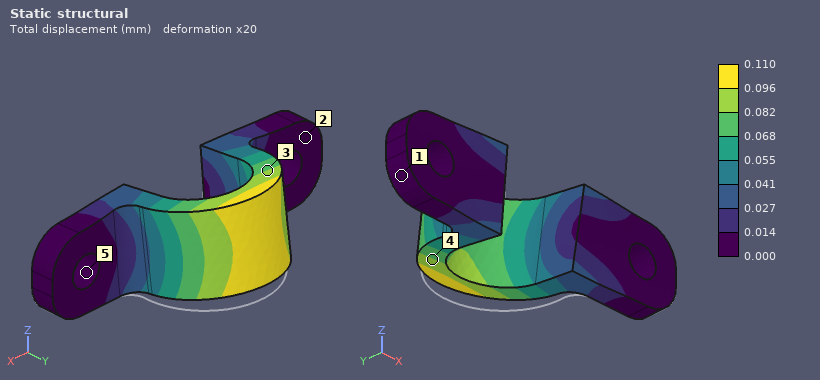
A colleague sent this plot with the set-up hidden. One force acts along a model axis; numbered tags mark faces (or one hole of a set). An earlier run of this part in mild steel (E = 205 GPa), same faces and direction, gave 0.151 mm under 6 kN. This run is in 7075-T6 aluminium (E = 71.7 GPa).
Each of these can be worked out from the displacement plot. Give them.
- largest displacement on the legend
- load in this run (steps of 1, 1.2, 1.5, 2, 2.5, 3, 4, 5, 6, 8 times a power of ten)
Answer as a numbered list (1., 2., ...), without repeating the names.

1. 0.110 mm
2. 1.5 kN
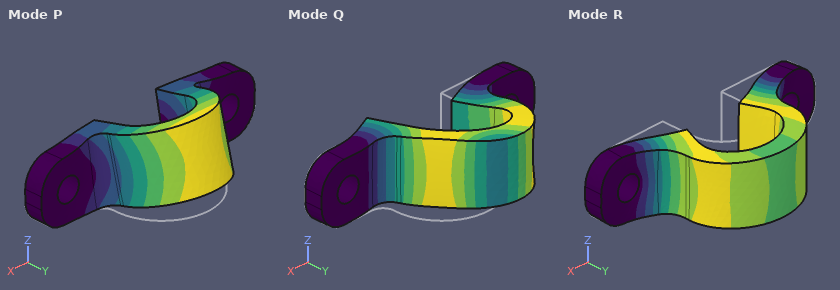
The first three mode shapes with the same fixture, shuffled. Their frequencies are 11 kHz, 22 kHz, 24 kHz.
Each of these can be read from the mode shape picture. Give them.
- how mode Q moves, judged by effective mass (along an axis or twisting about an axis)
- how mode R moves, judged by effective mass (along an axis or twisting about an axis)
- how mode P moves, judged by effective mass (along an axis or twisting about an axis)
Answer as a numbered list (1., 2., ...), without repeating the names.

1. along X
2. along Y
3. along Z
